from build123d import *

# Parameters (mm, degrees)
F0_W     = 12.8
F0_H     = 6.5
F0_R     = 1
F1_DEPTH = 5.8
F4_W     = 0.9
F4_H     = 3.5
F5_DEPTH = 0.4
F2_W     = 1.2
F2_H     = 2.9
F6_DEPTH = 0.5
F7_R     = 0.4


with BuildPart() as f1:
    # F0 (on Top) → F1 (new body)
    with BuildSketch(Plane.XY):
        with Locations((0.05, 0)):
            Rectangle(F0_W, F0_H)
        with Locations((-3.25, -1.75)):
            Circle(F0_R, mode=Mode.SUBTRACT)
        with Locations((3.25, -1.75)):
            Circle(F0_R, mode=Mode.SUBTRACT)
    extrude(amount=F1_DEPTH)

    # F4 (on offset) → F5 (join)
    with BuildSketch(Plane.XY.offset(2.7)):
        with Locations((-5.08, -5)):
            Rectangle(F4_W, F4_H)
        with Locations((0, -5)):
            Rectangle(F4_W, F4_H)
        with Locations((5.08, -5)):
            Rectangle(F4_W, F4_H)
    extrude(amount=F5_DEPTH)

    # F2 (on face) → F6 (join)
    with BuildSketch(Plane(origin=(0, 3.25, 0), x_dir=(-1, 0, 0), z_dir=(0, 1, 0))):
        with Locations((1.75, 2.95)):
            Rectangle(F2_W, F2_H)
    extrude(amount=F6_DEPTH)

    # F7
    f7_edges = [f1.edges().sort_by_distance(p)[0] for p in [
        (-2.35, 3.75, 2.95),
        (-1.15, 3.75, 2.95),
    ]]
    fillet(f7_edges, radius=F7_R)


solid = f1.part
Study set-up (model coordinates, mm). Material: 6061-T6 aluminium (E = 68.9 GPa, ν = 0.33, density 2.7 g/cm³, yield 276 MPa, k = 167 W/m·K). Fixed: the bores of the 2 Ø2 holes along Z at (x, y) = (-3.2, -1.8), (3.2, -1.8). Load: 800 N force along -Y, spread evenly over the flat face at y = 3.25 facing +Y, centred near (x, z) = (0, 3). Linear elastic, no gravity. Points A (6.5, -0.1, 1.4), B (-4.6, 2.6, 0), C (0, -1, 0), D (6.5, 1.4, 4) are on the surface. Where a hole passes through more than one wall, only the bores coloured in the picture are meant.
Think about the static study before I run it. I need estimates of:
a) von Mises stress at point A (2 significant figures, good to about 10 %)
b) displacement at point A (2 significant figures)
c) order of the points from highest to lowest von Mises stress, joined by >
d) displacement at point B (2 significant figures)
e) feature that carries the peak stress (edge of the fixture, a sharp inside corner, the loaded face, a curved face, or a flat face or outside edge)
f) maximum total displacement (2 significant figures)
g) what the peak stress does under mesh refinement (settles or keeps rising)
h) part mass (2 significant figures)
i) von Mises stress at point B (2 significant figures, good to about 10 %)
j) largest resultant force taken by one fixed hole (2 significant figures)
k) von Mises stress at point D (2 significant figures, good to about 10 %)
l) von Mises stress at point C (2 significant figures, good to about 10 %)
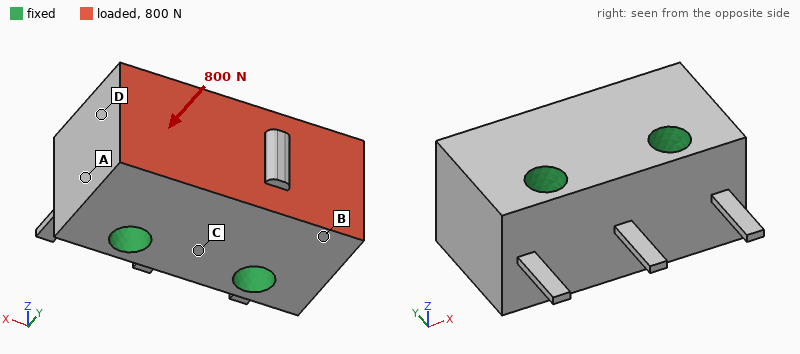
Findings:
5.3 MPa
0.75 µm
B > D > A > C
0.90 µm
edge of the fixture
1.3 µm
keeps rising
1.2 g
12 MPa
420 N
9.2 MPa
2.7 MPa
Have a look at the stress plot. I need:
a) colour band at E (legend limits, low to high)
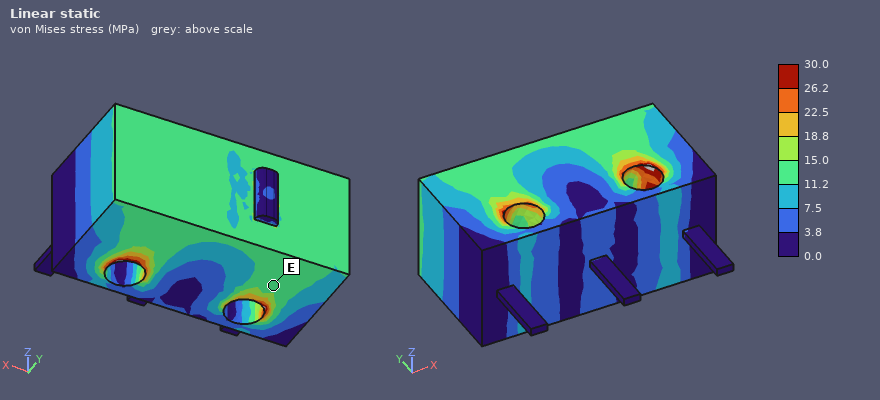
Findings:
11.2 to 15.0 MPa
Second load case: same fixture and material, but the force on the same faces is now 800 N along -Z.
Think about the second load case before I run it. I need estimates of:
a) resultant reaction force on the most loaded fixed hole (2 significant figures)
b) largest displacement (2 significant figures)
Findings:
410 N
5.7 µm
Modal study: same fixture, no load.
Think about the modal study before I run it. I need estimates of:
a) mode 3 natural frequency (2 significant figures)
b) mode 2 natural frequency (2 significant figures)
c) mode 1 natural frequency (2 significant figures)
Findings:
26 kHz
25 kHz
25 kHz
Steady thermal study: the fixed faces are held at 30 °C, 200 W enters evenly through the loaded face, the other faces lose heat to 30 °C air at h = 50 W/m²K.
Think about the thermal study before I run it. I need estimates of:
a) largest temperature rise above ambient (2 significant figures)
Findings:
81 K
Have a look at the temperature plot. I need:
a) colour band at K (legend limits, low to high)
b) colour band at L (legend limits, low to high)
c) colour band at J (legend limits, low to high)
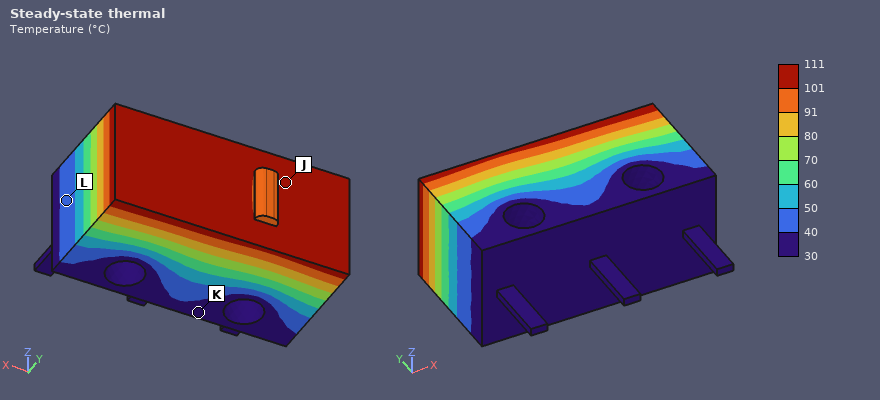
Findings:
30 to 40 °C
40 to 50 °C
101 to 111 °C
